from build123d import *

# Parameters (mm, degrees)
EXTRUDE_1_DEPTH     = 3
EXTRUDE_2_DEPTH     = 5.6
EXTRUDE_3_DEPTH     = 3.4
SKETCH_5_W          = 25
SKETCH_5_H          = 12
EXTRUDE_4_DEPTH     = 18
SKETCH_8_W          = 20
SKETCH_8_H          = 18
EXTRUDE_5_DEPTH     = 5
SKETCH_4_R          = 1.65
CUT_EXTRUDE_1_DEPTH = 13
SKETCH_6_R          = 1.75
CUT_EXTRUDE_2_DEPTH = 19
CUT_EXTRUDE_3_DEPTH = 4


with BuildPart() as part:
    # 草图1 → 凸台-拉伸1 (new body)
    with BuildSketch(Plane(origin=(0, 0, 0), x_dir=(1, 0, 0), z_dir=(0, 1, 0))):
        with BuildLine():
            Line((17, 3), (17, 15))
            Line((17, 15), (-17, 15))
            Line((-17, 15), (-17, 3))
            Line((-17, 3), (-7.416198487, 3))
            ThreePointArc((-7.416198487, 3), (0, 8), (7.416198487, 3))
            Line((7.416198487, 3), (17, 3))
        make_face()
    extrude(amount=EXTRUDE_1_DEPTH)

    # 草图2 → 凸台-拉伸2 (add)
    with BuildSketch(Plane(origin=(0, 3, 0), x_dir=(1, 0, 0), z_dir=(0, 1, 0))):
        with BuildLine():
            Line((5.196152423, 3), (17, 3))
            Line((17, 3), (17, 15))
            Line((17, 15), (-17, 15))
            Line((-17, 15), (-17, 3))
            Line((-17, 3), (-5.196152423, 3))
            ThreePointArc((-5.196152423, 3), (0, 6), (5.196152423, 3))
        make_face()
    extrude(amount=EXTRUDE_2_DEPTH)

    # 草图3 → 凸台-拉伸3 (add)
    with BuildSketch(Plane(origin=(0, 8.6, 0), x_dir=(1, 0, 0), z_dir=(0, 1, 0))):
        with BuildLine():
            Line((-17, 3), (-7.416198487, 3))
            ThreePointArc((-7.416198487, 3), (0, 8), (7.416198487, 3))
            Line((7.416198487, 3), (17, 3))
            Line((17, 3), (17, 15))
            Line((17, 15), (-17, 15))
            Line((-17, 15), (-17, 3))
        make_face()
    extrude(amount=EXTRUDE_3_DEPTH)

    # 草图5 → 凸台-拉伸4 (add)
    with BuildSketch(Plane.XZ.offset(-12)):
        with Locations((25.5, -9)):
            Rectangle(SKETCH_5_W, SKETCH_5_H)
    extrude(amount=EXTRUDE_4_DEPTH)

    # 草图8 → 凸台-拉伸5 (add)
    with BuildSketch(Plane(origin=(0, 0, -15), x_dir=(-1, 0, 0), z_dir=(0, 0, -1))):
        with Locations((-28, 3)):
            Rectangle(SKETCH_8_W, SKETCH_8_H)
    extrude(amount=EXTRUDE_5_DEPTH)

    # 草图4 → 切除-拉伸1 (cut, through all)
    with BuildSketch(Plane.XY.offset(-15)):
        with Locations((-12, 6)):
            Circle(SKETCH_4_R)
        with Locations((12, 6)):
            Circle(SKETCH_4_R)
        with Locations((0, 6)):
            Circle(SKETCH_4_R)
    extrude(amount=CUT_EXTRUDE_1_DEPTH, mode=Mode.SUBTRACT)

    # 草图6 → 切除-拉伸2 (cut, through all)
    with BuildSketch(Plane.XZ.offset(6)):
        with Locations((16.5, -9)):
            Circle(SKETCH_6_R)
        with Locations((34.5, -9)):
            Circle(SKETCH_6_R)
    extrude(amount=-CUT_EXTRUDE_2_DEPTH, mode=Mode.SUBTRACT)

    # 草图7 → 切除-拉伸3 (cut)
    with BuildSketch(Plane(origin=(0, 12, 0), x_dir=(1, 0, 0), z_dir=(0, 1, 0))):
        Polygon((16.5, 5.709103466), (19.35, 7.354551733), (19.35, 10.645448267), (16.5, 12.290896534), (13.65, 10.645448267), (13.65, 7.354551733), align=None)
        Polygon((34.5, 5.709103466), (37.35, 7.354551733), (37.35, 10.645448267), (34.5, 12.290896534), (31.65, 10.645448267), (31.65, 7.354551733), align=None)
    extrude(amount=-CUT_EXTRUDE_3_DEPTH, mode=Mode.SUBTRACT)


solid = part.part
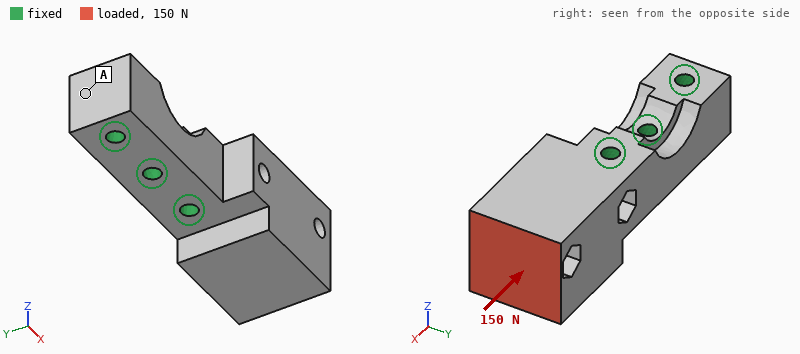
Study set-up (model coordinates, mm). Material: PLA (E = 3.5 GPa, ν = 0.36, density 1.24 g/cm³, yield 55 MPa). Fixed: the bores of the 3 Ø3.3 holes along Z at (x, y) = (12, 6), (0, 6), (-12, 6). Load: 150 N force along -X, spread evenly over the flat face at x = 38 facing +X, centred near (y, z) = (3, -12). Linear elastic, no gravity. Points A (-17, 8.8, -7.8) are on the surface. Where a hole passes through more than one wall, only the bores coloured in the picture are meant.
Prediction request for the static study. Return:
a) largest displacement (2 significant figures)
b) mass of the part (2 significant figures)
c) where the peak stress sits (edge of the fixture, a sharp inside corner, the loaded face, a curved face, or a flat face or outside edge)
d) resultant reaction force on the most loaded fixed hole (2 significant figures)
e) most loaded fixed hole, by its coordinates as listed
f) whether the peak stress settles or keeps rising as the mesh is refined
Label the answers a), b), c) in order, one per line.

a) 33 µm
b) 13 g
c) edge of the fixture
d) 130 N
e) (12, 6)
f) keeps rising
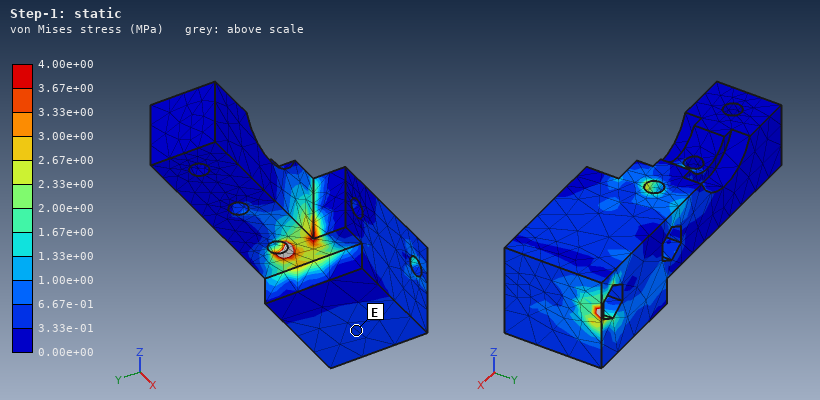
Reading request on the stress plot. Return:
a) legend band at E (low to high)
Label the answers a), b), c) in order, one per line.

a) 3.33e-01 to 6.67e-01 MPa
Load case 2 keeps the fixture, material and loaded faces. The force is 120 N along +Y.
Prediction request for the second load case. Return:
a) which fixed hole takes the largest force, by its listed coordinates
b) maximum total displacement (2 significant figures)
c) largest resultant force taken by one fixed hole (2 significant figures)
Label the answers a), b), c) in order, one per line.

a) (12, 6)
b) 0.20 mm
c) 260 N
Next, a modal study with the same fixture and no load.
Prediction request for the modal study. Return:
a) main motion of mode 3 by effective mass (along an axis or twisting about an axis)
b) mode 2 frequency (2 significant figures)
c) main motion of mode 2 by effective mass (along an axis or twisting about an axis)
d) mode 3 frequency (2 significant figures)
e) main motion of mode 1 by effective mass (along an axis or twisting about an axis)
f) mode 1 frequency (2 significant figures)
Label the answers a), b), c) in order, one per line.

a) twisting about X
b) 2900 Hz
c) along Z
d) 5200 Hz
e) along Y
f) 2300 Hz
